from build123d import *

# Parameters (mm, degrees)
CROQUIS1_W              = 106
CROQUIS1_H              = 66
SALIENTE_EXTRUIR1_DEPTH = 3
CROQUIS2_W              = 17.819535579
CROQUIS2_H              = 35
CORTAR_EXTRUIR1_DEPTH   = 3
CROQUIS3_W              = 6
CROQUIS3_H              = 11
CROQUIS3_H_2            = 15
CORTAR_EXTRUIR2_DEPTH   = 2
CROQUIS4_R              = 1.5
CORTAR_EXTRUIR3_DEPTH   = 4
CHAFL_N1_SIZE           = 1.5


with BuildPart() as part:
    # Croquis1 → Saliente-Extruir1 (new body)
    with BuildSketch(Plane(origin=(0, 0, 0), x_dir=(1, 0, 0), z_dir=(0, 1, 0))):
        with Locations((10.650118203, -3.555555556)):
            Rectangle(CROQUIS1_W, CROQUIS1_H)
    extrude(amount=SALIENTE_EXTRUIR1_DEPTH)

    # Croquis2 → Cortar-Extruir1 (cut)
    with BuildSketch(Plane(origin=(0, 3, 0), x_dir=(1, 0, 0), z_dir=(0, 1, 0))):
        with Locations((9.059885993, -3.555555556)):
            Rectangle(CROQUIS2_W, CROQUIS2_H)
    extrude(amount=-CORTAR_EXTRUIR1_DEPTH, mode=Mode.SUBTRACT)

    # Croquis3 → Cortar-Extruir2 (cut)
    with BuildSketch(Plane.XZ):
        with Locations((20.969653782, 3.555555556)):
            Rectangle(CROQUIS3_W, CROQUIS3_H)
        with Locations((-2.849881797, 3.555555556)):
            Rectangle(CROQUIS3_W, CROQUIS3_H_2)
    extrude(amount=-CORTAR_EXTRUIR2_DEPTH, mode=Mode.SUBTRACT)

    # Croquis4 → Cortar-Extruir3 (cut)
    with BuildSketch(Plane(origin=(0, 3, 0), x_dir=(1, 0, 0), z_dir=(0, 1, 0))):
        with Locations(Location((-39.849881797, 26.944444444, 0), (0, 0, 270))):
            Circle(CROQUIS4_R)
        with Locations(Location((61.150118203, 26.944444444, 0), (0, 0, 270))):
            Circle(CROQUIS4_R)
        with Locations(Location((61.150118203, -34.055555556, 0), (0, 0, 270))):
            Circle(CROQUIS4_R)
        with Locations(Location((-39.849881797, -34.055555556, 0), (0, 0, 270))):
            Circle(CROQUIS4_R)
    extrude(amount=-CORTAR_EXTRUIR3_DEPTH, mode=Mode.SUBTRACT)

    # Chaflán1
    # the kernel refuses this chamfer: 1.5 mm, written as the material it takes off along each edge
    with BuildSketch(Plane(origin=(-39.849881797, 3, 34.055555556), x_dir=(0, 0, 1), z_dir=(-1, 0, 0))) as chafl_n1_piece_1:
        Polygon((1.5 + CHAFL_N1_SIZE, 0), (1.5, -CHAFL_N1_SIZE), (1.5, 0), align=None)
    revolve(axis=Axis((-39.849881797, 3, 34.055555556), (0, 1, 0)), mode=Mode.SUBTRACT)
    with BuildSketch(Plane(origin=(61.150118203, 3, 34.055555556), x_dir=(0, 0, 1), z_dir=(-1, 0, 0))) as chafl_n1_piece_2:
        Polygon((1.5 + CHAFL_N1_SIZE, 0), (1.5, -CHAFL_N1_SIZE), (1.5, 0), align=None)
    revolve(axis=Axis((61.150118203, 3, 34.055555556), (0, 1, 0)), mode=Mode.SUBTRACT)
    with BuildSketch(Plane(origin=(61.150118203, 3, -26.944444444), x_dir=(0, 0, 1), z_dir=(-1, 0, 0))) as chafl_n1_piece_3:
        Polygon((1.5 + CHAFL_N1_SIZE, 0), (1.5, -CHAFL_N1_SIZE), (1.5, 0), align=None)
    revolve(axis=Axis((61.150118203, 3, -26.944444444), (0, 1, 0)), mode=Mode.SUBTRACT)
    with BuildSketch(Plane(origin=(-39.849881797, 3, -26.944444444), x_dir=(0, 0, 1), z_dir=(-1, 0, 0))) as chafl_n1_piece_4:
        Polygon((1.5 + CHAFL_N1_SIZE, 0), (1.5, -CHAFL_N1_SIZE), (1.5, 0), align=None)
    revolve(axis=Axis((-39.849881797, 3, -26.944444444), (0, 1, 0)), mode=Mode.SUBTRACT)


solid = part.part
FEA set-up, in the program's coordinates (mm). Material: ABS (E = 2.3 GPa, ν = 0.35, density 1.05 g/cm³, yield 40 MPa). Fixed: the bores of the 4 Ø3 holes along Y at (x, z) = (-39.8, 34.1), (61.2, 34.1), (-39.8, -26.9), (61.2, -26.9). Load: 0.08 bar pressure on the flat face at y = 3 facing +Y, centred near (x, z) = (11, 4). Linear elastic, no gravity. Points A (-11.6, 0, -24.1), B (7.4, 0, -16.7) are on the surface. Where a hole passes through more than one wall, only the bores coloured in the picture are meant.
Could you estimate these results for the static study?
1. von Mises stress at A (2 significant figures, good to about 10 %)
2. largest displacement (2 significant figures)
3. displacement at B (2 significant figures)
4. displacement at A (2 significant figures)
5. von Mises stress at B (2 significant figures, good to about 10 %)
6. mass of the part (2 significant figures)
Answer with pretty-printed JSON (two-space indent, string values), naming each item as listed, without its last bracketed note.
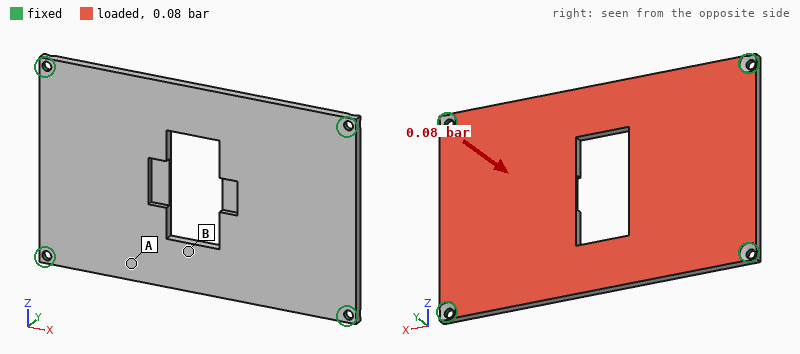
{
  "von Mises stress at A": "1.8 MPa",
  "largest displacement": "1.2 mm",
  "displacement at B": "1.1 mm",
  "displacement at A": "0.73 mm",
  "von Mises stress at B": "4.7 MPa",
  "mass of the part": "20 g"
}
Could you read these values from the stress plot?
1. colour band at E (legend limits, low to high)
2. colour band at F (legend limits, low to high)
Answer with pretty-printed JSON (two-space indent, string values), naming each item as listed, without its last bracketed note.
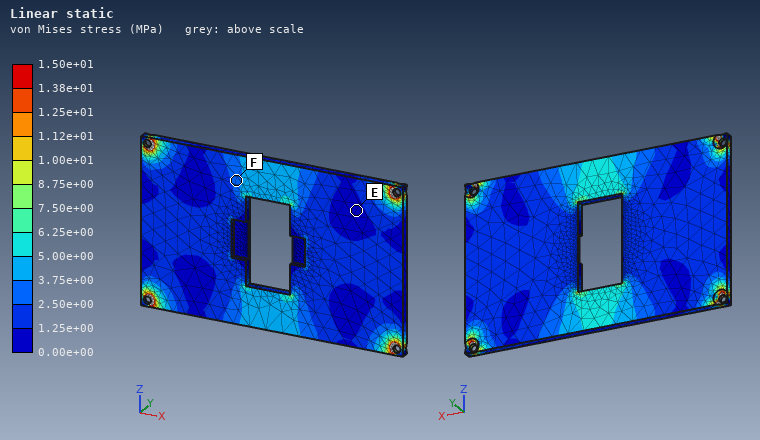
{
  "colour band at E": "0.00e+00 to 1.25e+00 MPa",
  "colour band at F": "2.50e+00 to 3.75e+00 MPa"
}
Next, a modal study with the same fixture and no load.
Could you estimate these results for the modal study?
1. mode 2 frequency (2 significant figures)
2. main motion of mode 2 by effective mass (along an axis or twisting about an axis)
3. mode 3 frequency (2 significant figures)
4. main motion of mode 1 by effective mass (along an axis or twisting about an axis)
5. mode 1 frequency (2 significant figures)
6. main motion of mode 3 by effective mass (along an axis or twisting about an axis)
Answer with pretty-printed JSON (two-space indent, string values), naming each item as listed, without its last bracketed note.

{
  "mode 2 frequency": "560 Hz",
  "main motion of mode 2 by effective mass": "twisting about X",
  "mode 3 frequency": "740 Hz",
  "main motion of mode 1 by effective mass": "along Y",
  "mode 1 frequency": "290 Hz",
  "main motion of mode 3 by effective mass": "twisting about Z"
}
